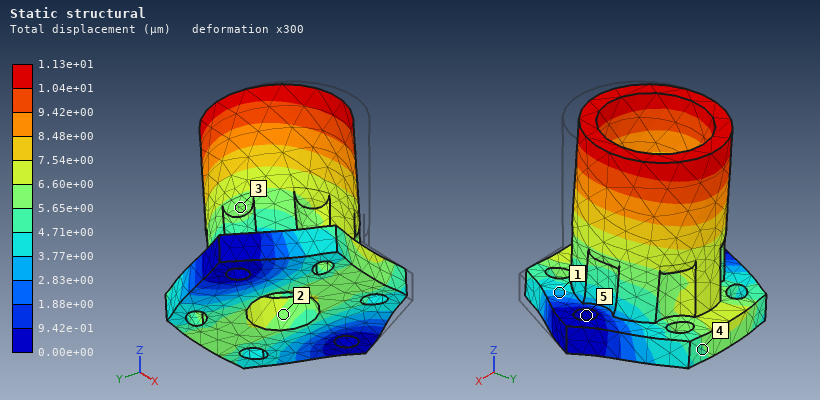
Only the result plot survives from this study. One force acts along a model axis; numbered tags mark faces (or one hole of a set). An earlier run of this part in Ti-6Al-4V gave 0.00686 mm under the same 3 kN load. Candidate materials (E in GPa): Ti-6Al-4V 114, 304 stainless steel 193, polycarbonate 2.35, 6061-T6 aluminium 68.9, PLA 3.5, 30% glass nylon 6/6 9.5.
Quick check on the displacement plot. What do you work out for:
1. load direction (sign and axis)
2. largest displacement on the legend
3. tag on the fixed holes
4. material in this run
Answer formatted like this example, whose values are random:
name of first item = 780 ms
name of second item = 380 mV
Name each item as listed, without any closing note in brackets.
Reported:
load direction = +Y
largest displacement on the legend = 1.13e+01 µm
tag on the fixed holes = 5
material in this run = 6061-T6 aluminium
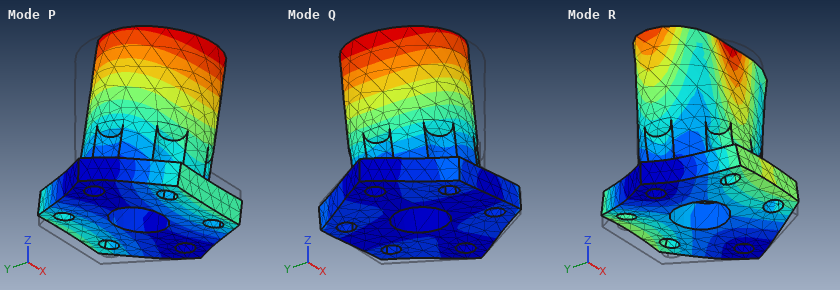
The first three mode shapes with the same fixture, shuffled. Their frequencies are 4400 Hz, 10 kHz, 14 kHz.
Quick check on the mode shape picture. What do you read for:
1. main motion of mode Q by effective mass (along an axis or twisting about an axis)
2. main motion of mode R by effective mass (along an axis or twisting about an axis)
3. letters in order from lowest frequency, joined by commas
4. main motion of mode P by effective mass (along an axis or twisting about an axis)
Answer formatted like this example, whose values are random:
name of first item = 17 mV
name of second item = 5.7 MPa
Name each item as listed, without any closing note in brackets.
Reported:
main motion of mode Q by effective mass = along X
main motion of mode R by effective mass = along Z
letters in order from lowest frequency, joined by commas = P, Q, R
main motion of mode P by effective mass = along Y
